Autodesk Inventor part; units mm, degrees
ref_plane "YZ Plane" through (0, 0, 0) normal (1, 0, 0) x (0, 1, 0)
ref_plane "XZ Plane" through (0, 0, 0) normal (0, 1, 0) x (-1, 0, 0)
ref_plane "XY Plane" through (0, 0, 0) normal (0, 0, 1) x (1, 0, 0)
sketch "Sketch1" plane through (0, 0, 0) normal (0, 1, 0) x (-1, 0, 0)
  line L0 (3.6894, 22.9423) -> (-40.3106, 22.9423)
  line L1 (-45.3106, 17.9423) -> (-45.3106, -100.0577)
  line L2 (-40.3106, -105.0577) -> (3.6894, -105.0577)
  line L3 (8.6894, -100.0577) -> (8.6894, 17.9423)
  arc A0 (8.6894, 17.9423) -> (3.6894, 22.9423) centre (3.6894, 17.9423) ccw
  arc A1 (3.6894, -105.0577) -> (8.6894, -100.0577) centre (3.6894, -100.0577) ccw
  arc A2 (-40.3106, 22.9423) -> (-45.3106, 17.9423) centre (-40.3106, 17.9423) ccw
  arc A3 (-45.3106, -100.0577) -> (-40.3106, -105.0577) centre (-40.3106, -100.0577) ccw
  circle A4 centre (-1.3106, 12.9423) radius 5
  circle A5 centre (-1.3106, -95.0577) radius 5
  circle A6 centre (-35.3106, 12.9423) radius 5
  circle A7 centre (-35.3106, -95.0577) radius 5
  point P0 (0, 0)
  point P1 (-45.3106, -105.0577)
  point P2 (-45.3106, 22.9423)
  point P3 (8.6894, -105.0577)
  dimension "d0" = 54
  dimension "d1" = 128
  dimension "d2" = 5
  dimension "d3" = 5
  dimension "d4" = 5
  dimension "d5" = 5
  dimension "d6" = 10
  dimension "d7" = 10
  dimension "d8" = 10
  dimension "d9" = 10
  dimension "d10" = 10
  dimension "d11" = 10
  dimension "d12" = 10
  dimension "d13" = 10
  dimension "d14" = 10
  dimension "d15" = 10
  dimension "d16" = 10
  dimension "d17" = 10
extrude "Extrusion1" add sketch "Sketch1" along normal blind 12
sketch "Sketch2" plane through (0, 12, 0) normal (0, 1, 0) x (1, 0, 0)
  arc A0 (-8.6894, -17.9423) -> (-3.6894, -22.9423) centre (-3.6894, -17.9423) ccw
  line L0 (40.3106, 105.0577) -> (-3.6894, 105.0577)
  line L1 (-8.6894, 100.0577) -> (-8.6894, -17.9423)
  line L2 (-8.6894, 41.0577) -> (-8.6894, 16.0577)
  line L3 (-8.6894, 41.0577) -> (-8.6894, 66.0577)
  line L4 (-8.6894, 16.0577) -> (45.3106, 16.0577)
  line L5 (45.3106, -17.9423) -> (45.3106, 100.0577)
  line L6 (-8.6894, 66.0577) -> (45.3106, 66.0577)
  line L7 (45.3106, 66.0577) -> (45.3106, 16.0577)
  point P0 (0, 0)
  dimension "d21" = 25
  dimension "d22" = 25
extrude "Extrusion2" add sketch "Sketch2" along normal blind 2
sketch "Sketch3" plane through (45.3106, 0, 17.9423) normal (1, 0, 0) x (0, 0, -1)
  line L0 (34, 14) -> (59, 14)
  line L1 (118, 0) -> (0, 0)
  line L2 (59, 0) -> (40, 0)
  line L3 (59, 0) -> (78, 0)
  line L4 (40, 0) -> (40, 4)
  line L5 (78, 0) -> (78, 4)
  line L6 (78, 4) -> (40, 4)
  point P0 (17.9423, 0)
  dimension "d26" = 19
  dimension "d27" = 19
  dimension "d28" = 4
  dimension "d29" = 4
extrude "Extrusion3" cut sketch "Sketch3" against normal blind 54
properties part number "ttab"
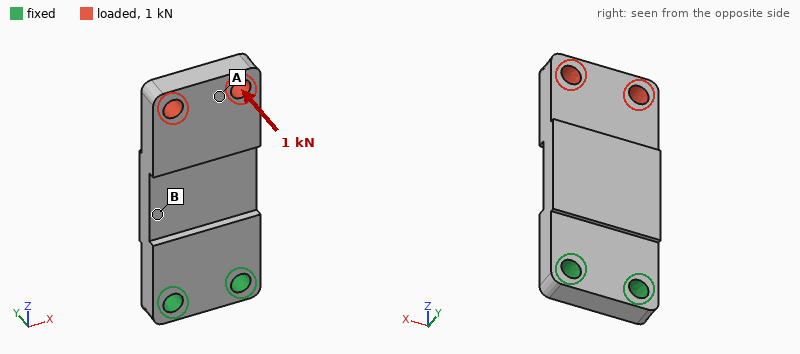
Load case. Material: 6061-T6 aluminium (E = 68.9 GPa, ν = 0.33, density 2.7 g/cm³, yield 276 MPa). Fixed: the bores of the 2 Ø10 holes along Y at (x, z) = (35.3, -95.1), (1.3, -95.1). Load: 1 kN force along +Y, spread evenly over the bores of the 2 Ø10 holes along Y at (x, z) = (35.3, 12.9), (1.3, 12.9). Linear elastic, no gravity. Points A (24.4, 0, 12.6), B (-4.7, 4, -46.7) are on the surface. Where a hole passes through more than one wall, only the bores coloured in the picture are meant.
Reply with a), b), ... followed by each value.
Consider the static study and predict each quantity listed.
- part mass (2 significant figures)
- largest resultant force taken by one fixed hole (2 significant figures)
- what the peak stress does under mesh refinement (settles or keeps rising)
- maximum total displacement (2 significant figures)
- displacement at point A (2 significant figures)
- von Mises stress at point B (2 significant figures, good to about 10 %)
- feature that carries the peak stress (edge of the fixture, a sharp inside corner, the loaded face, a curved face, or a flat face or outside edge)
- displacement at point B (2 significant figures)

a) 210 g
b) 510 N
c) keeps rising
d) 1.1 mm
e) 0.92 mm
f) 64 MPa
g) edge of the fixture
h) 0.19 mm
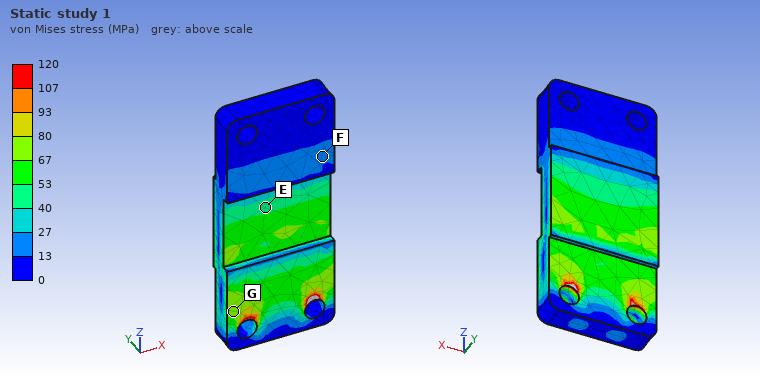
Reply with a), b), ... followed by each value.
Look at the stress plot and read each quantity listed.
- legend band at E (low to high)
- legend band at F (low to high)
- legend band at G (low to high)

a) 40 to 53 MPa
b) 13 to 27 MPa
c) 67 to 80 MPa
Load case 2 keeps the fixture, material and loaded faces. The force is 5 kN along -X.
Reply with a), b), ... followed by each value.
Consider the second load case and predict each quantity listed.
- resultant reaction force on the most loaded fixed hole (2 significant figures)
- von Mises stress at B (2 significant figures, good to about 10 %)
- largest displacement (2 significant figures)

a) 14 kN
b) 68 MPa
c) 0.32 mm
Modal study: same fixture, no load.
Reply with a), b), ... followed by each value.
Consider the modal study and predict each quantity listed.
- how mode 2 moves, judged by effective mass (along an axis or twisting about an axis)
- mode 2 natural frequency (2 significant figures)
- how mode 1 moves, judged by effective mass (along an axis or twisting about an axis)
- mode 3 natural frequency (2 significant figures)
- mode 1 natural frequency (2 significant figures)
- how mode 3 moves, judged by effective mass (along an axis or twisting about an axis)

a) along X
b) 2600 Hz
c) along Y
d) 3100 Hz
e) 700 Hz
f) along X
